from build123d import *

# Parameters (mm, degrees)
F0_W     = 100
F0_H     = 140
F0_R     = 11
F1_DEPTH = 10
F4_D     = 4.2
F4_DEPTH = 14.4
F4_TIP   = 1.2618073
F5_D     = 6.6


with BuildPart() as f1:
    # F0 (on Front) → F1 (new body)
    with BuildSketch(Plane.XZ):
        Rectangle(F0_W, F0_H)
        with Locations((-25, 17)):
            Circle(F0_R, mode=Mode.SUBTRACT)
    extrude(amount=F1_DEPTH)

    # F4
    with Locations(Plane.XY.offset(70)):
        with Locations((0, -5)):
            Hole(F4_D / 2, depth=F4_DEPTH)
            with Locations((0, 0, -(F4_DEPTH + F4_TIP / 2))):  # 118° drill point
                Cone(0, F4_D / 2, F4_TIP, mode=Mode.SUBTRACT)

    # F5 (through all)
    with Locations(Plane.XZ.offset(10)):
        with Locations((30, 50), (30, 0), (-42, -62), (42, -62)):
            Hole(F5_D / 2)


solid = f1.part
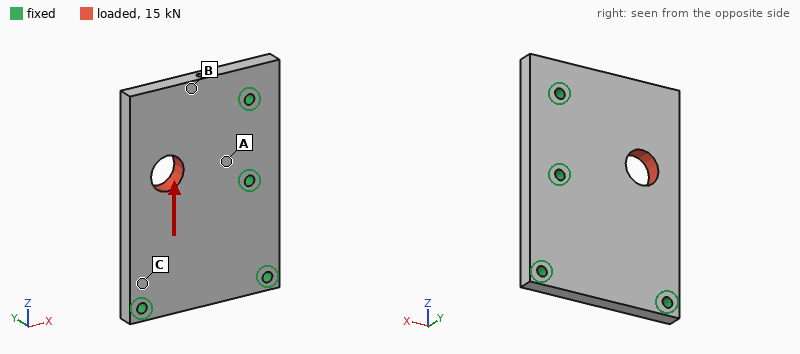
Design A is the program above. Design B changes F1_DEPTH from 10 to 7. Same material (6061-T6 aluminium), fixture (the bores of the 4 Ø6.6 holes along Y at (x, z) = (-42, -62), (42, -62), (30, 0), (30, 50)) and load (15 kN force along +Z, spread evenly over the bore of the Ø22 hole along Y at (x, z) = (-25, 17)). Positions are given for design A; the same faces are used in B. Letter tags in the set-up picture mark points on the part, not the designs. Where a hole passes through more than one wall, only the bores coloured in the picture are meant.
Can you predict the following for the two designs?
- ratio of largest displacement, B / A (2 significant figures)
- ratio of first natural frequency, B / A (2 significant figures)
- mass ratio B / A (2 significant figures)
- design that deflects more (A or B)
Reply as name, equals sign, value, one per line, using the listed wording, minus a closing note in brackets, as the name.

ratio of largest displacement, B / A = 1.5
ratio of first natural frequency, B / A = 0.72
mass ratio B / A = 0.70
design that deflects more = B
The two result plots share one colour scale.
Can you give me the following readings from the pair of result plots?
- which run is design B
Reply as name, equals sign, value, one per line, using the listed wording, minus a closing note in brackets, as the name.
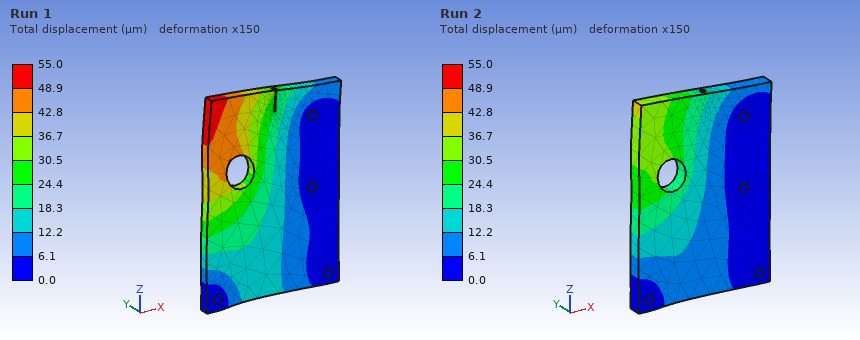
which run is design B = Run 1
